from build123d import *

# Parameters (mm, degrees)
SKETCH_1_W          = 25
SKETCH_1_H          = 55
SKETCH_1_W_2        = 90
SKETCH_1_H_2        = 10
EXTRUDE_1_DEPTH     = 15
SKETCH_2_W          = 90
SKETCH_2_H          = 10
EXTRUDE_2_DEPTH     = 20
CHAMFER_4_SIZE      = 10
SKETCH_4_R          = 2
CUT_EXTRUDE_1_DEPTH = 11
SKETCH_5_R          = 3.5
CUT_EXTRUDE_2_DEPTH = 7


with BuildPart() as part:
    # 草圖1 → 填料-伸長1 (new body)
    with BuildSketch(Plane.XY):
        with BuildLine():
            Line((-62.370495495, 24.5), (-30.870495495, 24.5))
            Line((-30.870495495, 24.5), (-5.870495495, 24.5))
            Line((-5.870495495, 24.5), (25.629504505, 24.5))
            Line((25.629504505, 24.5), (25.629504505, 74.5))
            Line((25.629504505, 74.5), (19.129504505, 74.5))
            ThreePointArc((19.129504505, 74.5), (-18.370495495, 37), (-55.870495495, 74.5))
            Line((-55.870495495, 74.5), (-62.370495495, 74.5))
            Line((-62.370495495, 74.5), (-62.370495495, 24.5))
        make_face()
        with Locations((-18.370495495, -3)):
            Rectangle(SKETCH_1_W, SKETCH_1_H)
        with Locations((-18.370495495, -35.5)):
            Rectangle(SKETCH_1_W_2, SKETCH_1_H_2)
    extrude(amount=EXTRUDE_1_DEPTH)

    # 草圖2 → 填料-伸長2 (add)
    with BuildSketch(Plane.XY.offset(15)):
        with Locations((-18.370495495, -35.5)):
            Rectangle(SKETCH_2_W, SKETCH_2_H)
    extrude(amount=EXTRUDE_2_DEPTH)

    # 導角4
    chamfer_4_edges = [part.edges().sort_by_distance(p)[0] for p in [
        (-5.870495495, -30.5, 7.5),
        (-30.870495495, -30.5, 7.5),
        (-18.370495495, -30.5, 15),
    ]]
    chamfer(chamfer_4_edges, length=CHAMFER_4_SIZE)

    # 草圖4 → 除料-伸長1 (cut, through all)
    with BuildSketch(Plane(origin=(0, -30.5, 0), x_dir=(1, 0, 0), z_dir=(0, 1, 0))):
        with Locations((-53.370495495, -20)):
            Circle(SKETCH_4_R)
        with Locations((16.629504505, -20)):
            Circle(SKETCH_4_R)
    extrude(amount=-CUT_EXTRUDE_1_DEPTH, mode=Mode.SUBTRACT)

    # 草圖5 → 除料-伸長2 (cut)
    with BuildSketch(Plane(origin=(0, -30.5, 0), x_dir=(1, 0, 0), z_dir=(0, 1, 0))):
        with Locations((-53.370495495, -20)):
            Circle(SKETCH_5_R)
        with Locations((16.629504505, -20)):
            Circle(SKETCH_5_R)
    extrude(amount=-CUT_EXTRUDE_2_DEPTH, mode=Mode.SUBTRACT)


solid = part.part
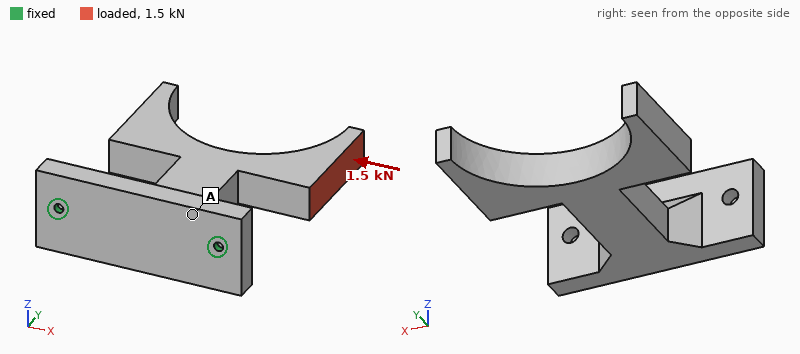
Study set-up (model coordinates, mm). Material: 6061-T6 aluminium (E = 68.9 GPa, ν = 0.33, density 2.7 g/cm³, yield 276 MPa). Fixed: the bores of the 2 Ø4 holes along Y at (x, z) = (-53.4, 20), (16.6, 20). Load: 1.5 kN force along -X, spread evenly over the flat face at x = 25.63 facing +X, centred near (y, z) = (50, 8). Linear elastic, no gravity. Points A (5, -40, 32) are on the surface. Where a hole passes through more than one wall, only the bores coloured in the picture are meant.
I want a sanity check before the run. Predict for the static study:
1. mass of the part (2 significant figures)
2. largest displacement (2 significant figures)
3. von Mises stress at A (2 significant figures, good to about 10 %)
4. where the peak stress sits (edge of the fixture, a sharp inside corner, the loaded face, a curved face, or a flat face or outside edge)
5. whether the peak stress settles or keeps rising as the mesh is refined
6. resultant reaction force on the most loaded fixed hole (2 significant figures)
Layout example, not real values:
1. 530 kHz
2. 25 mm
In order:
1. 240 g
2. 0.55 mm
3. 20 MPa
4. edge of the fixture
5. keeps rising
6. 2.1 kN
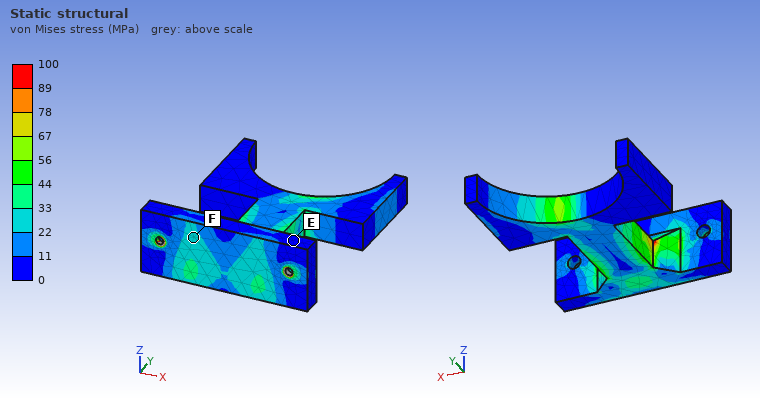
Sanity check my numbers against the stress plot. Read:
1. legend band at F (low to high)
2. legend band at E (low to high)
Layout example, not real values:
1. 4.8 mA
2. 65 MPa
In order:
1. 22 to 33 MPa
2. 0 to 11 MPa
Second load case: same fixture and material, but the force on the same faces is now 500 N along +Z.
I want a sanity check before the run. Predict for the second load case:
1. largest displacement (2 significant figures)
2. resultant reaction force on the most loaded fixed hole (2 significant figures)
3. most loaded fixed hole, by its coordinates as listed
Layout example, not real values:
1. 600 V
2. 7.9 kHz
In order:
1. 1.6 mm
2. 570 N
3. (16.6, 20)
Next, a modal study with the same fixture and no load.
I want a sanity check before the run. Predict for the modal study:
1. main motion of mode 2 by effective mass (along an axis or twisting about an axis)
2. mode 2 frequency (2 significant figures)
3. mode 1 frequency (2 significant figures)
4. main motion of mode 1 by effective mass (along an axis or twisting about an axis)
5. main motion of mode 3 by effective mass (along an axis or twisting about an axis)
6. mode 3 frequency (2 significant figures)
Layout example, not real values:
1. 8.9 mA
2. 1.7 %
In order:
1. along X
2. 1200 Hz
3. 380 Hz
4. along Z
5. twisting about Y
6. 1400 Hz
